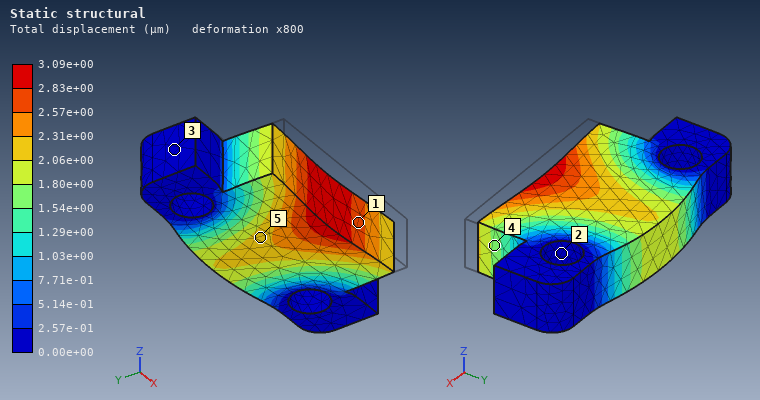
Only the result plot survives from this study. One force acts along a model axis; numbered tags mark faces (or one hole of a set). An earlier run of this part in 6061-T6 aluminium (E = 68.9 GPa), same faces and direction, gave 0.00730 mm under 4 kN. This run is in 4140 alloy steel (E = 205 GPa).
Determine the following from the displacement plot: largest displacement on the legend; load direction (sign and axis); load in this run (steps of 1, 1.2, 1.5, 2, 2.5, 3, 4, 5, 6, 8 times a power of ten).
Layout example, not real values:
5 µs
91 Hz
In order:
3.09e+00 µm
+Y
5 kN
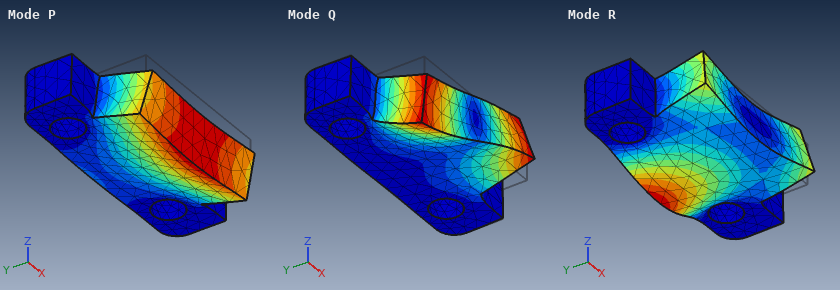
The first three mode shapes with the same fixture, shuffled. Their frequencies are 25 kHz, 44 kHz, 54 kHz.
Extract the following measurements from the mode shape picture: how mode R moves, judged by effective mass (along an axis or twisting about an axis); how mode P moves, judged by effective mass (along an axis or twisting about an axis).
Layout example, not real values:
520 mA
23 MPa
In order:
along Z
along Z
